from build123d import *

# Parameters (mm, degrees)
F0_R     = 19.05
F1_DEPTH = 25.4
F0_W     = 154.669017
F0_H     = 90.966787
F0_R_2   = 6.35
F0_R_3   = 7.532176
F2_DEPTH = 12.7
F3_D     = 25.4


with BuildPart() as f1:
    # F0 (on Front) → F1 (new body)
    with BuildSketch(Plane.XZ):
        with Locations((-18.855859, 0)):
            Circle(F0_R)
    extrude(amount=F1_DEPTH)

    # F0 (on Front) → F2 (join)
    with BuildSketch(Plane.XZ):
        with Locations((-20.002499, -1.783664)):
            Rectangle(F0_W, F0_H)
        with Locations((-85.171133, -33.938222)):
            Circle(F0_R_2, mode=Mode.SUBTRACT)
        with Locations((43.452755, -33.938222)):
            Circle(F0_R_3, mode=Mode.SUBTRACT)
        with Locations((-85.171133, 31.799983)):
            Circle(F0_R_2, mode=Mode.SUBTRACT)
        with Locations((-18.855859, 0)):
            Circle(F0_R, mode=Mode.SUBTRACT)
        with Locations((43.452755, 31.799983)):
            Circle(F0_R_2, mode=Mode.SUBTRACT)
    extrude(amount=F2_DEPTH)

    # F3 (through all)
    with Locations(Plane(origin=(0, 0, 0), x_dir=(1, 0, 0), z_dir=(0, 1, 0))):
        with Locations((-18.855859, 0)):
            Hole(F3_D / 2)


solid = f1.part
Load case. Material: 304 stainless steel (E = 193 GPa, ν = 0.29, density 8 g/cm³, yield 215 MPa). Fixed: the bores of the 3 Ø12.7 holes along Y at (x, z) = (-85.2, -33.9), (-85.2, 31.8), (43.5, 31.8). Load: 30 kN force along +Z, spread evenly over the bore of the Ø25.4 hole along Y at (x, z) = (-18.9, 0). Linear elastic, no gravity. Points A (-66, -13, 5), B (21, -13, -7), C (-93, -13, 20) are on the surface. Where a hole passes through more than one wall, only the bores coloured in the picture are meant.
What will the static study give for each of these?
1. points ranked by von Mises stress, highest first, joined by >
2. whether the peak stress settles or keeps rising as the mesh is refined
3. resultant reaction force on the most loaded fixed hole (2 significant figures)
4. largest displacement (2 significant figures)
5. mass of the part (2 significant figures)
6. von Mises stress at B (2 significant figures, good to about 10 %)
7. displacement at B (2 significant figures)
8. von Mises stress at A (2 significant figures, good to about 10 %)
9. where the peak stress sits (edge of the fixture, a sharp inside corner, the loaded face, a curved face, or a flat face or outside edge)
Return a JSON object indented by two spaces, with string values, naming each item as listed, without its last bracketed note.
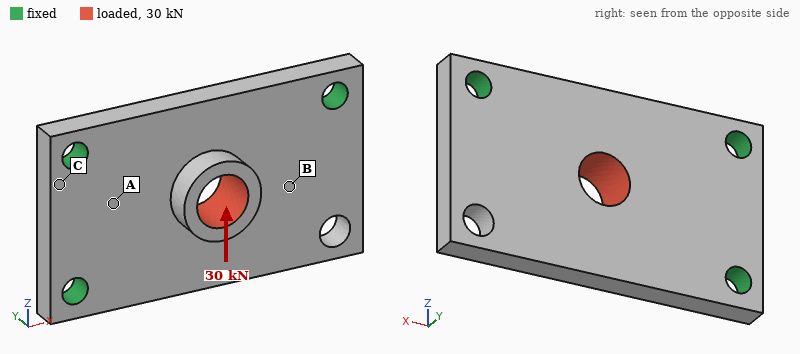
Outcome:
{
  "points ranked by von Mises stress, highest first, joined by >": "A > B > C",
  "whether the peak stress settles or keeps rising as the mesh is refined": "keeps rising",
  "resultant reaction force on the most loaded fixed hole": "14 kN",
  "largest displacement": "59 µm",
  "mass of the part": "1.4 kg",
  "von Mises stress at B": "33 MPa",
  "displacement at B": "25 µm",
  "von Mises stress at A": "55 MPa",
  "where the peak stress sits": "edge of the fixture"
}
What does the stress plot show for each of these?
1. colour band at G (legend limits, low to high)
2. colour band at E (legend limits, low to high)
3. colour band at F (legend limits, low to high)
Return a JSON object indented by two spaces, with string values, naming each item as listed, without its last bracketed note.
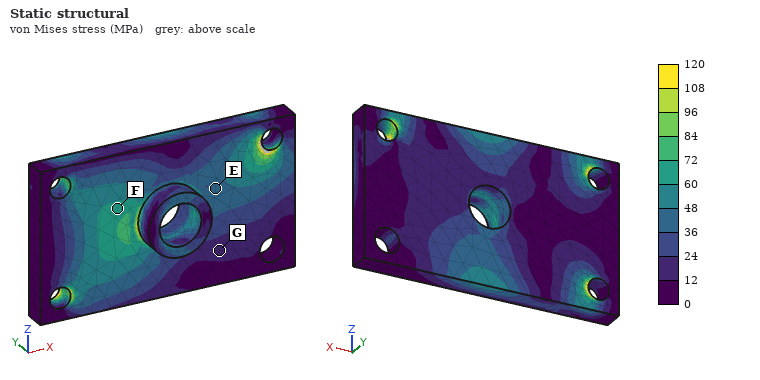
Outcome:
{
  "colour band at G": "12 to 24 MPa",
  "colour band at E": "36 to 48 MPa",
  "colour band at F": "60 to 72 MPa"
}
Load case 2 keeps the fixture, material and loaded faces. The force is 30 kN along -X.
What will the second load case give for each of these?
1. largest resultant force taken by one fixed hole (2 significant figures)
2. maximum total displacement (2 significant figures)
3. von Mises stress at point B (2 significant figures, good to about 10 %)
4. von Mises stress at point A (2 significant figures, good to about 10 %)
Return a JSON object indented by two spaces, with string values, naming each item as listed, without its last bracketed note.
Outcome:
{
  "largest resultant force taken by one fixed hole": "11 kN",
  "maximum total displacement": "29 µm",
  "von Mises stress at point B": "21 MPa",
  "von Mises stress at point A": "19 MPa"
}
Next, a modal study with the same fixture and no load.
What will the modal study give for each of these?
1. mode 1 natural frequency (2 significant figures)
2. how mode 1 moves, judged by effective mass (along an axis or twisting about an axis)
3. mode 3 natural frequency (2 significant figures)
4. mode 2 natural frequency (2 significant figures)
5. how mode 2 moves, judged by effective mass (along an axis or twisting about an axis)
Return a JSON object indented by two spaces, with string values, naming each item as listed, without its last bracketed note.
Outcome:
{
  "mode 1 natural frequency": "2000 Hz",
  "how mode 1 moves, judged by effective mass": "along Y",
  "mode 3 natural frequency": "5200 Hz",
  "mode 2 natural frequency": "3700 Hz",
  "how mode 2 moves, judged by effective mass": "along Y"
}
